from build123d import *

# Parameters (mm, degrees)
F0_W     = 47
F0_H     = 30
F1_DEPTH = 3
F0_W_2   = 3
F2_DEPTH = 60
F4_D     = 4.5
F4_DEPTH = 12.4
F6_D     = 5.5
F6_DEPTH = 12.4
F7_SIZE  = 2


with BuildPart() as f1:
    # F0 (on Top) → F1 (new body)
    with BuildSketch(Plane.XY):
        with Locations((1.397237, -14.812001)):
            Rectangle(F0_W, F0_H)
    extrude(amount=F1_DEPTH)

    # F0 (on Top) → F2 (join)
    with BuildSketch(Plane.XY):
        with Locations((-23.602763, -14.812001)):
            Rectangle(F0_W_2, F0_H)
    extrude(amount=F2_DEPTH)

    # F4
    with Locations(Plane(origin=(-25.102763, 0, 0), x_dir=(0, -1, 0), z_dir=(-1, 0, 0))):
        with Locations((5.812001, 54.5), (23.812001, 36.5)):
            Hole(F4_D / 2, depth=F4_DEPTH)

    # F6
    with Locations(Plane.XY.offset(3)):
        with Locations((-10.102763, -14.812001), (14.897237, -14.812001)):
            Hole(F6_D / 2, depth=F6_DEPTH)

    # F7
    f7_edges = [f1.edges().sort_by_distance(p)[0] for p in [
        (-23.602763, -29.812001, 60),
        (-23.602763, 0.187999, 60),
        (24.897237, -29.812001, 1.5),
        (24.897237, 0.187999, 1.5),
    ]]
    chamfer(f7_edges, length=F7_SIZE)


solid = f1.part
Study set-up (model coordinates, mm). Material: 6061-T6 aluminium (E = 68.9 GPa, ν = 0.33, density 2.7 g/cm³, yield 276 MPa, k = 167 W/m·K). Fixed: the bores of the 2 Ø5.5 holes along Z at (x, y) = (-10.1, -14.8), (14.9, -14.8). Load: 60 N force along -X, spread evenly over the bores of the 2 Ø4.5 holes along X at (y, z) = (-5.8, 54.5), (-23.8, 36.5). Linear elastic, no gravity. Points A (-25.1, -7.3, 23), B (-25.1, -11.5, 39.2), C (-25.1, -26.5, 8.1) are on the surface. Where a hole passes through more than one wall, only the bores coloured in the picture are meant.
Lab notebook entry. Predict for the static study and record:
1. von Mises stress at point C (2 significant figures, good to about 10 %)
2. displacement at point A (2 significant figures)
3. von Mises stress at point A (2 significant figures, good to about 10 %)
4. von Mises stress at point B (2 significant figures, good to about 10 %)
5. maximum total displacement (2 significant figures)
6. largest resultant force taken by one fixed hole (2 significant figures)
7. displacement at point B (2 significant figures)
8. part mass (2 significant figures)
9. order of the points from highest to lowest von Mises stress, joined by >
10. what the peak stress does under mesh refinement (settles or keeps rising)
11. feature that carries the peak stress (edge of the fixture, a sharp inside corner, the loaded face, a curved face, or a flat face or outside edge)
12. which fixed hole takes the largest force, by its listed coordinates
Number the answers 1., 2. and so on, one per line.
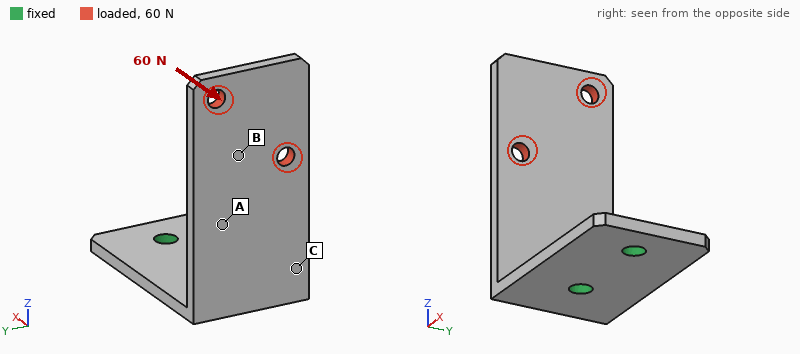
1. 48 MPa
2. 0.25 mm
3. 29 MPa
4. 13 MPa
5. 0.93 mm
6. 61 N
7. 0.53 mm
8. 25 g
9. C > A > B
10. keeps rising
11. edge of the fixture
12. (-10.1, -14.8)
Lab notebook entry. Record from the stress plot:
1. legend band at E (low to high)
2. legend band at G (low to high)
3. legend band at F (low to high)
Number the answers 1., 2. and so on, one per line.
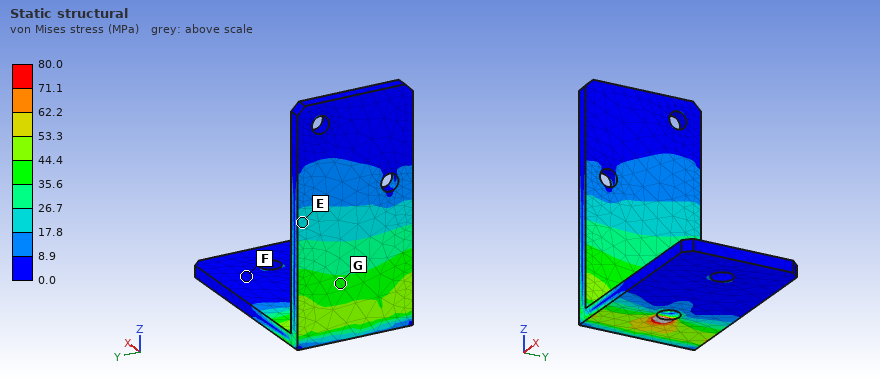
1. 17.8 to 26.7 MPa
2. 35.6 to 44.4 MPa
3. 0.0 to 8.9 MPa
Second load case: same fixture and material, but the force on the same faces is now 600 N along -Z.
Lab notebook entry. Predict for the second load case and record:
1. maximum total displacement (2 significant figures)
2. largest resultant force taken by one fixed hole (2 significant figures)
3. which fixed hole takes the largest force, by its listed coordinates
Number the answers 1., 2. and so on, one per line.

1. 0.64 mm
2. 660 N
3. (-10.1, -14.8)
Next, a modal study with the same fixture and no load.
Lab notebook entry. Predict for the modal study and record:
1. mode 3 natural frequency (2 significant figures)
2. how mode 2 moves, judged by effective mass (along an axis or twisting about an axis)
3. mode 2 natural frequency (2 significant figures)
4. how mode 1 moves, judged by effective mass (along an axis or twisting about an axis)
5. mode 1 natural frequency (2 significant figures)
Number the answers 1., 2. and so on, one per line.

1. 2900 Hz
2. along Y
3. 1000 Hz
4. along X
5. 550 Hz
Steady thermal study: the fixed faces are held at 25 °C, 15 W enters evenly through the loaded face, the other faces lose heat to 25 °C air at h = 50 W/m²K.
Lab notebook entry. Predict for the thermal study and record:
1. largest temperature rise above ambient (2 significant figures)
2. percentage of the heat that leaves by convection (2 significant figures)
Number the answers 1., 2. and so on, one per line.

1. 46 K
2. 38 %
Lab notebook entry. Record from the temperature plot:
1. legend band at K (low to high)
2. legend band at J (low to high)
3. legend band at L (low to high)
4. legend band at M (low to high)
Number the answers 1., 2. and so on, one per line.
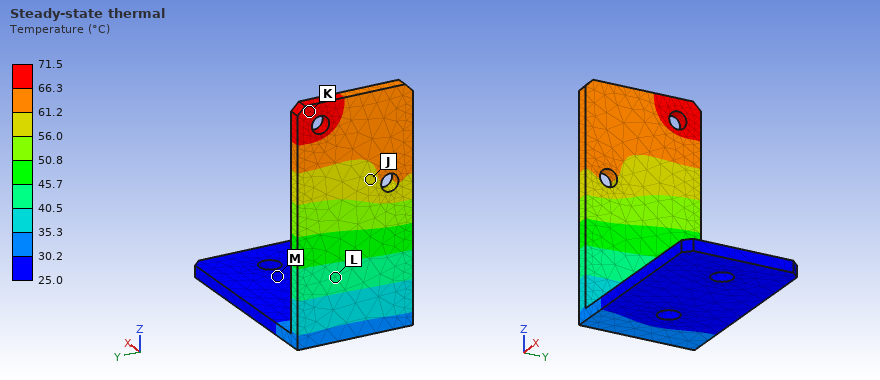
1. 66.3 to 71.5 °C
2. 56.0 to 61.2 °C
3. 40.5 to 45.7 °C
4. 25.0 to 30.2 °C
